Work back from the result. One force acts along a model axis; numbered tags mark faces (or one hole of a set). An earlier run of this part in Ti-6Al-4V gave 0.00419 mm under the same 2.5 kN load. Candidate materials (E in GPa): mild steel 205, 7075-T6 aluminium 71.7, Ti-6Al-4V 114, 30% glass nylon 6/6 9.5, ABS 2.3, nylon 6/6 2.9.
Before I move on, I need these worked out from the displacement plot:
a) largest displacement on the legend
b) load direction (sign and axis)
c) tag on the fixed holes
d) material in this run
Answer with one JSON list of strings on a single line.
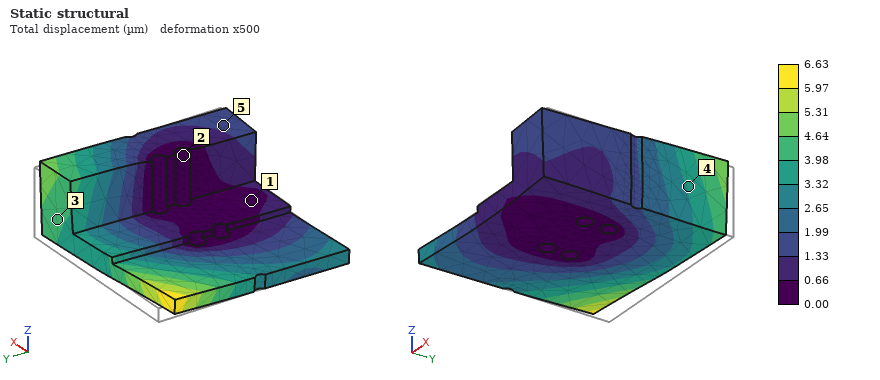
["6.63 µm", "-Y", "2", "7075-T6 aluminium"]
